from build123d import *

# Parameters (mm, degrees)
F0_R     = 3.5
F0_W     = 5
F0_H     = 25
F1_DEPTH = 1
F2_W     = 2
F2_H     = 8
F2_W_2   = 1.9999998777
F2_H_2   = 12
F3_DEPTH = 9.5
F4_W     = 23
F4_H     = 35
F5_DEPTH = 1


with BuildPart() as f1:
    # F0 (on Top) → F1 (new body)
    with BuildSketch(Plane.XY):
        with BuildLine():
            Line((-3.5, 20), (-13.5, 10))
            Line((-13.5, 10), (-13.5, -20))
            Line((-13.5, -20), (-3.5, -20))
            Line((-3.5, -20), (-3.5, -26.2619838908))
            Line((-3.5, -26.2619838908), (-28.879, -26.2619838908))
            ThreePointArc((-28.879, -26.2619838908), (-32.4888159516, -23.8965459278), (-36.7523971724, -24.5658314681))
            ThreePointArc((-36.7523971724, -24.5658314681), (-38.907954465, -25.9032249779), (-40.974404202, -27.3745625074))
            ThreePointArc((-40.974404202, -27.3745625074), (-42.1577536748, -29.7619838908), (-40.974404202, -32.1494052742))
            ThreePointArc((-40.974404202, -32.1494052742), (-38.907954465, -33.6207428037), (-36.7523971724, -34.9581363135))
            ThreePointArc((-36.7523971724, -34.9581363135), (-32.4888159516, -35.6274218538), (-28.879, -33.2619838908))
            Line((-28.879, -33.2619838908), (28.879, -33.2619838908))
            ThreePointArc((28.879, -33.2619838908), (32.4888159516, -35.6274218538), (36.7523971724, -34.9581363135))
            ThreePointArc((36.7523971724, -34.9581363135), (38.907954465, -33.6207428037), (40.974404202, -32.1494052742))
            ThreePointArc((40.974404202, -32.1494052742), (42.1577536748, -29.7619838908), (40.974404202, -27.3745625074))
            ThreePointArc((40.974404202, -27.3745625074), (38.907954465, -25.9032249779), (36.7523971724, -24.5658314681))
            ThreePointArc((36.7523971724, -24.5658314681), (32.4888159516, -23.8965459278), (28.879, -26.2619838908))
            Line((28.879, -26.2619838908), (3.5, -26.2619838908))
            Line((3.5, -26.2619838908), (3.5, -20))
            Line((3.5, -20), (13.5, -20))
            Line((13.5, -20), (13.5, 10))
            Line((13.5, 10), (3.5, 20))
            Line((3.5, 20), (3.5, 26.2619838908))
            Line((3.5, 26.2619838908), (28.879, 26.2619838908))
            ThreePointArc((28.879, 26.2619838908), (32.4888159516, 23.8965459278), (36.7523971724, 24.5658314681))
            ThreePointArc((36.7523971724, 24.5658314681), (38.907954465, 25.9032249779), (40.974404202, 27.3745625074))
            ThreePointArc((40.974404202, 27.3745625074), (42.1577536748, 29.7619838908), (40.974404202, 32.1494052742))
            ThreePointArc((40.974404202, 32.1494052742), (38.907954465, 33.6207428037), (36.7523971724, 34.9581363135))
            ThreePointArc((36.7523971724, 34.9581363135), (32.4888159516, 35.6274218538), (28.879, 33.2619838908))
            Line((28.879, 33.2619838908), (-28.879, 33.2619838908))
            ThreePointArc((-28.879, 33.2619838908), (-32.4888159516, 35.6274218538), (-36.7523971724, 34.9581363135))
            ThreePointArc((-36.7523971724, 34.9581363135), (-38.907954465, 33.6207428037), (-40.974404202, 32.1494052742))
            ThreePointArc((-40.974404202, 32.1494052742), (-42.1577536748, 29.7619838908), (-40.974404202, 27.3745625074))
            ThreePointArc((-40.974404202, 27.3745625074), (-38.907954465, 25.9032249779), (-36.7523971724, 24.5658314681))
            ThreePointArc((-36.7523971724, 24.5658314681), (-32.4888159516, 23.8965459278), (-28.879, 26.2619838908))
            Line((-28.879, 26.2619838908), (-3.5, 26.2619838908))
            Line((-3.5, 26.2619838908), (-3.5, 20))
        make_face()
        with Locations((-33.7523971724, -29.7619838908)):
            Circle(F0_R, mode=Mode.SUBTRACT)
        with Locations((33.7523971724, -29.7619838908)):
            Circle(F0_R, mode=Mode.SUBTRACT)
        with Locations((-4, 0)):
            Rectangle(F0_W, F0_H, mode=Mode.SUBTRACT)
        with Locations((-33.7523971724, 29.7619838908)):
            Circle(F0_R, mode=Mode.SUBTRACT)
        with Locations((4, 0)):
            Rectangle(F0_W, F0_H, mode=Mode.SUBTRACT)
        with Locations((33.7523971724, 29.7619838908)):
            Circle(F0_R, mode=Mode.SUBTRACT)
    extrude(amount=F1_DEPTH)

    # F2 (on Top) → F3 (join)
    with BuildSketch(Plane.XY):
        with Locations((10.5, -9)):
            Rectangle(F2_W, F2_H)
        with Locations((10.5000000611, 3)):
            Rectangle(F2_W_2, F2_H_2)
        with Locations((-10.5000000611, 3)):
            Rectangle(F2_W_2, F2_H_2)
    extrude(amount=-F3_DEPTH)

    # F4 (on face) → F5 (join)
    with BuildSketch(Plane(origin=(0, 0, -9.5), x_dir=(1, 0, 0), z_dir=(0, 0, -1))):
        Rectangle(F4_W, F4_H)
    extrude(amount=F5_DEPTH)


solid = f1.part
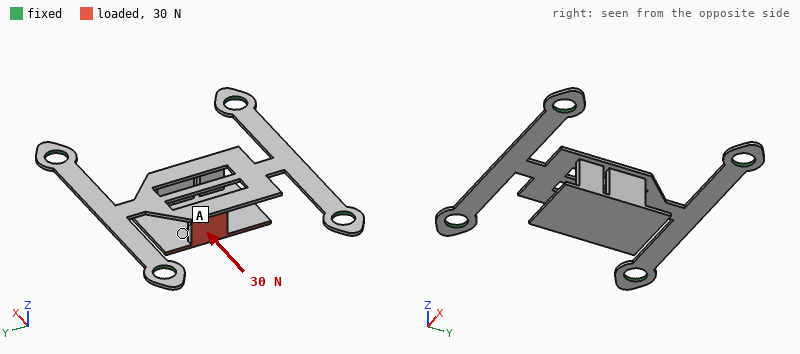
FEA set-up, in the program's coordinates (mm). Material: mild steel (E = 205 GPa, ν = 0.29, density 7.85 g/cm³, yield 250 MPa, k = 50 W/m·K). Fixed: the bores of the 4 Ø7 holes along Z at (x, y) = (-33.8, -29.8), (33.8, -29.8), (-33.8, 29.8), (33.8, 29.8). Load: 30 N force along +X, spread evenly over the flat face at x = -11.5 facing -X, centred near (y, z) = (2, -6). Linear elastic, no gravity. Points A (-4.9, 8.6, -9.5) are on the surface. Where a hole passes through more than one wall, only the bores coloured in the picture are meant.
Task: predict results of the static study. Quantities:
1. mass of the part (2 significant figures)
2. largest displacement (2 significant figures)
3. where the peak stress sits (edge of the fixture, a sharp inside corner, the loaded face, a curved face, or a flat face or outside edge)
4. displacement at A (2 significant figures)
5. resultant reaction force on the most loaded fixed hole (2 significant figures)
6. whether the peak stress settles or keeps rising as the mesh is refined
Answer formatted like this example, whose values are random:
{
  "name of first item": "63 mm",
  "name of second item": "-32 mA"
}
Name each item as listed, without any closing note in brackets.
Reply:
{
  "mass of the part": "26 g",
  "largest displacement": "0.17 mm",
  "where the peak stress sits": "a sharp inside corner",
  "displacement at A": "0.11 mm",
  "resultant reaction force on the most loaded fixed hole": "9.0 N",
  "whether the peak stress settles or keeps rising as the mesh is refined": "keeps rising"
}
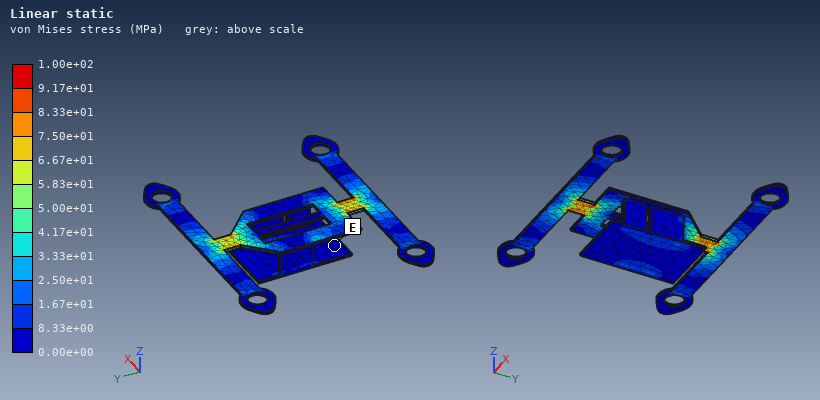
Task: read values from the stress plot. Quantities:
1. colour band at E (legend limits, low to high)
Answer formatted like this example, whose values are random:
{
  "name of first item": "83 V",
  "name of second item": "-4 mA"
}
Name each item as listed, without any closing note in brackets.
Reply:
{
  "colour band at E": "0.00e+00 to 8.33e+00 MPa"
}
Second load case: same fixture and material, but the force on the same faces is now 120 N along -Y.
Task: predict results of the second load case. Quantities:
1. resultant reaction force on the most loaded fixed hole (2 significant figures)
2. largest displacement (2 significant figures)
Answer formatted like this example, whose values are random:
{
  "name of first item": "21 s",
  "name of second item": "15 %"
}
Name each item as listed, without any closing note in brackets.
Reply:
{
  "resultant reaction force on the most loaded fixed hole": "39 N",
  "largest displacement": "0.26 mm"
}
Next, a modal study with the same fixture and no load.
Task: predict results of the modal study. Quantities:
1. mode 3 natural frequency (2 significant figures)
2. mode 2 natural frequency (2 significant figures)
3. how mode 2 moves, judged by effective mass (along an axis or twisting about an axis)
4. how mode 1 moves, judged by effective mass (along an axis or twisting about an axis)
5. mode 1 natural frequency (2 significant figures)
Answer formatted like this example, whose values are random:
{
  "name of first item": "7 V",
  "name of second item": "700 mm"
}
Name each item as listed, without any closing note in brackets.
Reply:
{
  "mode 3 natural frequency": "800 Hz",
  "mode 2 natural frequency": "510 Hz",
  "how mode 2 moves, judged by effective mass": "along X",
  "how mode 1 moves, judged by effective mass": "along Z",
  "mode 1 natural frequency": "400 Hz"
}
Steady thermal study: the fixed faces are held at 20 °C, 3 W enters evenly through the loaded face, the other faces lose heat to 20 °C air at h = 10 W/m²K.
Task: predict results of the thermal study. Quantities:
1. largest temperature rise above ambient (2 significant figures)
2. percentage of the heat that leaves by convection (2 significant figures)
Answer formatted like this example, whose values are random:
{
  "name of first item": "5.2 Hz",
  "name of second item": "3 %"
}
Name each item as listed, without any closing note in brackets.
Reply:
{
  "largest temperature rise above ambient": "66 K",
  "percentage of the heat that leaves by convection": "70 %"
}
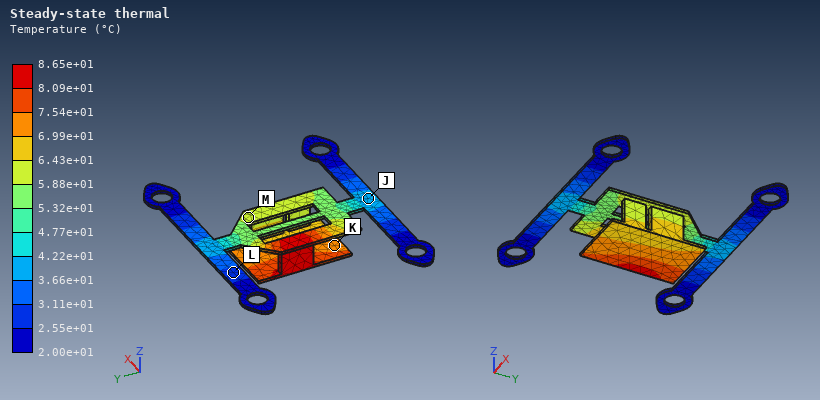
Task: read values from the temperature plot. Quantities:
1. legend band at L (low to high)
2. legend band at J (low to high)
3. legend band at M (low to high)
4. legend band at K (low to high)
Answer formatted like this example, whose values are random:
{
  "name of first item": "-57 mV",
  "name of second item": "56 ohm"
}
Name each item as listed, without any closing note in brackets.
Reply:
{
  "legend band at L": "2.55e+01 to 3.11e+01 °C",
  "legend band at J": "3.66e+01 to 4.22e+01 °C",
  "legend band at M": "5.88e+01 to 6.43e+01 °C",
  "legend band at K": "6.99e+01 to 7.54e+01 °C"
}
